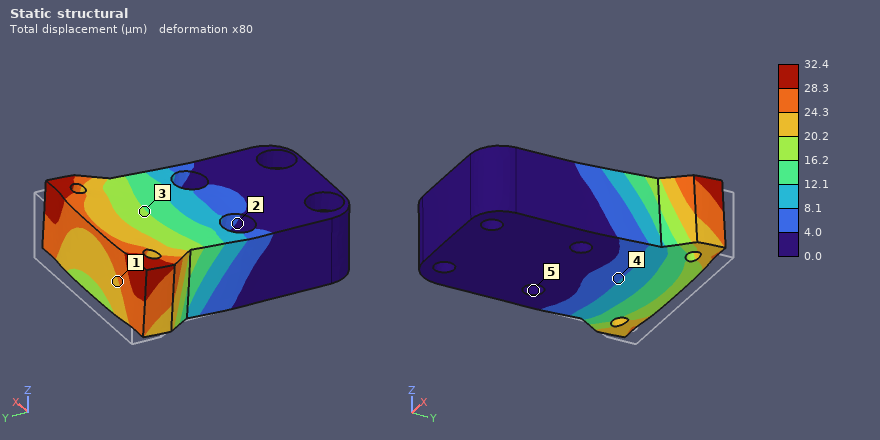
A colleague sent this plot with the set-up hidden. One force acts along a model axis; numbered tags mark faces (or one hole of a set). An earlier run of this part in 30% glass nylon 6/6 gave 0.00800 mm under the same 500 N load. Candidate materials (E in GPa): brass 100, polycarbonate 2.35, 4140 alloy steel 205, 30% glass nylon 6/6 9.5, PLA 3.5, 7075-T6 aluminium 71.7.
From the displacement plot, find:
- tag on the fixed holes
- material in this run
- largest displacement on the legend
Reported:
5
polycarbonate
32.4 µm
